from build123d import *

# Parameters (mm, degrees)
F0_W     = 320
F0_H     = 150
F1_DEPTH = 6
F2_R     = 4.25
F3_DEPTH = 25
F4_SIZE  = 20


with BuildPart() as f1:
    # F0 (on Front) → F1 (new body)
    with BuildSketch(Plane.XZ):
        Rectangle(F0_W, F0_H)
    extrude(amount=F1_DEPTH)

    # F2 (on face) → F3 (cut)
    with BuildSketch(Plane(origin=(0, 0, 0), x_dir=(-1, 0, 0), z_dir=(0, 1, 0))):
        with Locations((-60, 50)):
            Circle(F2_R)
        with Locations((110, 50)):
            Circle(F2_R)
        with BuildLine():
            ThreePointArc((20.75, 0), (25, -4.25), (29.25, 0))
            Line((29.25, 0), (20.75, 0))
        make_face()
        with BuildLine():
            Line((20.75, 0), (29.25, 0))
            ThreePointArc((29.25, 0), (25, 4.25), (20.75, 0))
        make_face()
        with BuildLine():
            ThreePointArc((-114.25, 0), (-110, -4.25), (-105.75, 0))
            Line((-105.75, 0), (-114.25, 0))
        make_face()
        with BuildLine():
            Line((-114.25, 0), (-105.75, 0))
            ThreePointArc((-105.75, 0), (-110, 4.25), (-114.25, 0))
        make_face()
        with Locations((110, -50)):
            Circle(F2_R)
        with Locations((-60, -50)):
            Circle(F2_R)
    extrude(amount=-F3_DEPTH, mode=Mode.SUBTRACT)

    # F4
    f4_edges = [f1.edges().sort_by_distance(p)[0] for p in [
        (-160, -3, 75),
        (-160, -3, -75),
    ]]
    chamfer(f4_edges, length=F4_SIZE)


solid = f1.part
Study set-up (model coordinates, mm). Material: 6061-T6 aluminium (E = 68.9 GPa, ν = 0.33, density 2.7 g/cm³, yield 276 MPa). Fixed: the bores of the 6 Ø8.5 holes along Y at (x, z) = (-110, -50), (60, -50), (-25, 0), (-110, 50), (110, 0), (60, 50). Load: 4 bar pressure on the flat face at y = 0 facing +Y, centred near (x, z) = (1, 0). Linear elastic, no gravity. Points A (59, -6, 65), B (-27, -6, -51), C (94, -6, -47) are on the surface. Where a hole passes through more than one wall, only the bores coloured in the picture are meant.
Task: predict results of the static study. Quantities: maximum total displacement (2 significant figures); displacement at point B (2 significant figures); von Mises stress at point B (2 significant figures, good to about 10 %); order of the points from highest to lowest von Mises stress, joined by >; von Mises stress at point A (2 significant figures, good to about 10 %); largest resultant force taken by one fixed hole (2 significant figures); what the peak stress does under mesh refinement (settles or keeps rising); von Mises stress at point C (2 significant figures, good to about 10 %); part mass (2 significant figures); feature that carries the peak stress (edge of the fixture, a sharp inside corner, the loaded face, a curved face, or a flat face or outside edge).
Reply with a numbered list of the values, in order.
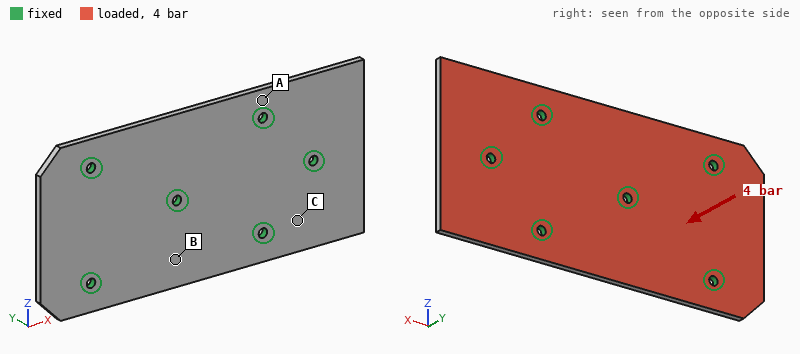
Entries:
1. 0.96 mm
2. 0.25 mm
3. 19 MPa
4. A > C > B
5. 72 MPa
6. 4.0 kN
7. keeps rising
8. 47 MPa
9. 770 g
10. edge of the fixture
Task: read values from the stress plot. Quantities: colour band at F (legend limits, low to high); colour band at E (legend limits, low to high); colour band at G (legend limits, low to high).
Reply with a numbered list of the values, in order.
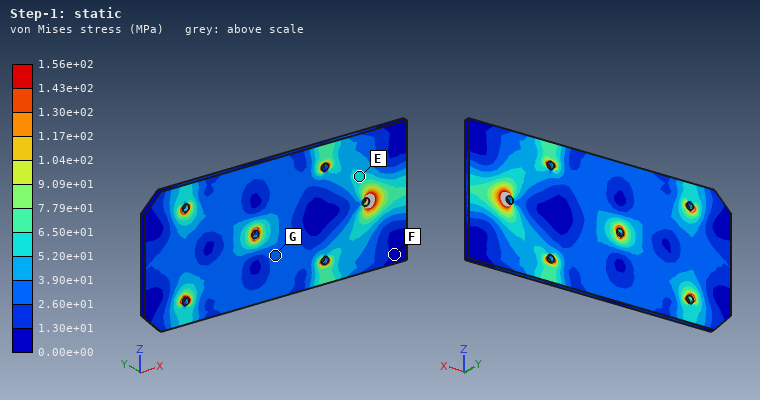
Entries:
1. 0.00e+00 to 1.30e+01 MPa
2. 5.20e+01 to 6.50e+01 MPa
3. 2.60e+01 to 3.90e+01 MPa
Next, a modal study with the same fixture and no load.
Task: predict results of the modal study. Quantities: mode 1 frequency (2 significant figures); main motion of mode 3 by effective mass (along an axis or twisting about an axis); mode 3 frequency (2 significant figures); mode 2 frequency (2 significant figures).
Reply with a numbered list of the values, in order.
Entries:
1. 1000 Hz
2. twisting about X
3. 1500 Hz
4. 1100 Hz
